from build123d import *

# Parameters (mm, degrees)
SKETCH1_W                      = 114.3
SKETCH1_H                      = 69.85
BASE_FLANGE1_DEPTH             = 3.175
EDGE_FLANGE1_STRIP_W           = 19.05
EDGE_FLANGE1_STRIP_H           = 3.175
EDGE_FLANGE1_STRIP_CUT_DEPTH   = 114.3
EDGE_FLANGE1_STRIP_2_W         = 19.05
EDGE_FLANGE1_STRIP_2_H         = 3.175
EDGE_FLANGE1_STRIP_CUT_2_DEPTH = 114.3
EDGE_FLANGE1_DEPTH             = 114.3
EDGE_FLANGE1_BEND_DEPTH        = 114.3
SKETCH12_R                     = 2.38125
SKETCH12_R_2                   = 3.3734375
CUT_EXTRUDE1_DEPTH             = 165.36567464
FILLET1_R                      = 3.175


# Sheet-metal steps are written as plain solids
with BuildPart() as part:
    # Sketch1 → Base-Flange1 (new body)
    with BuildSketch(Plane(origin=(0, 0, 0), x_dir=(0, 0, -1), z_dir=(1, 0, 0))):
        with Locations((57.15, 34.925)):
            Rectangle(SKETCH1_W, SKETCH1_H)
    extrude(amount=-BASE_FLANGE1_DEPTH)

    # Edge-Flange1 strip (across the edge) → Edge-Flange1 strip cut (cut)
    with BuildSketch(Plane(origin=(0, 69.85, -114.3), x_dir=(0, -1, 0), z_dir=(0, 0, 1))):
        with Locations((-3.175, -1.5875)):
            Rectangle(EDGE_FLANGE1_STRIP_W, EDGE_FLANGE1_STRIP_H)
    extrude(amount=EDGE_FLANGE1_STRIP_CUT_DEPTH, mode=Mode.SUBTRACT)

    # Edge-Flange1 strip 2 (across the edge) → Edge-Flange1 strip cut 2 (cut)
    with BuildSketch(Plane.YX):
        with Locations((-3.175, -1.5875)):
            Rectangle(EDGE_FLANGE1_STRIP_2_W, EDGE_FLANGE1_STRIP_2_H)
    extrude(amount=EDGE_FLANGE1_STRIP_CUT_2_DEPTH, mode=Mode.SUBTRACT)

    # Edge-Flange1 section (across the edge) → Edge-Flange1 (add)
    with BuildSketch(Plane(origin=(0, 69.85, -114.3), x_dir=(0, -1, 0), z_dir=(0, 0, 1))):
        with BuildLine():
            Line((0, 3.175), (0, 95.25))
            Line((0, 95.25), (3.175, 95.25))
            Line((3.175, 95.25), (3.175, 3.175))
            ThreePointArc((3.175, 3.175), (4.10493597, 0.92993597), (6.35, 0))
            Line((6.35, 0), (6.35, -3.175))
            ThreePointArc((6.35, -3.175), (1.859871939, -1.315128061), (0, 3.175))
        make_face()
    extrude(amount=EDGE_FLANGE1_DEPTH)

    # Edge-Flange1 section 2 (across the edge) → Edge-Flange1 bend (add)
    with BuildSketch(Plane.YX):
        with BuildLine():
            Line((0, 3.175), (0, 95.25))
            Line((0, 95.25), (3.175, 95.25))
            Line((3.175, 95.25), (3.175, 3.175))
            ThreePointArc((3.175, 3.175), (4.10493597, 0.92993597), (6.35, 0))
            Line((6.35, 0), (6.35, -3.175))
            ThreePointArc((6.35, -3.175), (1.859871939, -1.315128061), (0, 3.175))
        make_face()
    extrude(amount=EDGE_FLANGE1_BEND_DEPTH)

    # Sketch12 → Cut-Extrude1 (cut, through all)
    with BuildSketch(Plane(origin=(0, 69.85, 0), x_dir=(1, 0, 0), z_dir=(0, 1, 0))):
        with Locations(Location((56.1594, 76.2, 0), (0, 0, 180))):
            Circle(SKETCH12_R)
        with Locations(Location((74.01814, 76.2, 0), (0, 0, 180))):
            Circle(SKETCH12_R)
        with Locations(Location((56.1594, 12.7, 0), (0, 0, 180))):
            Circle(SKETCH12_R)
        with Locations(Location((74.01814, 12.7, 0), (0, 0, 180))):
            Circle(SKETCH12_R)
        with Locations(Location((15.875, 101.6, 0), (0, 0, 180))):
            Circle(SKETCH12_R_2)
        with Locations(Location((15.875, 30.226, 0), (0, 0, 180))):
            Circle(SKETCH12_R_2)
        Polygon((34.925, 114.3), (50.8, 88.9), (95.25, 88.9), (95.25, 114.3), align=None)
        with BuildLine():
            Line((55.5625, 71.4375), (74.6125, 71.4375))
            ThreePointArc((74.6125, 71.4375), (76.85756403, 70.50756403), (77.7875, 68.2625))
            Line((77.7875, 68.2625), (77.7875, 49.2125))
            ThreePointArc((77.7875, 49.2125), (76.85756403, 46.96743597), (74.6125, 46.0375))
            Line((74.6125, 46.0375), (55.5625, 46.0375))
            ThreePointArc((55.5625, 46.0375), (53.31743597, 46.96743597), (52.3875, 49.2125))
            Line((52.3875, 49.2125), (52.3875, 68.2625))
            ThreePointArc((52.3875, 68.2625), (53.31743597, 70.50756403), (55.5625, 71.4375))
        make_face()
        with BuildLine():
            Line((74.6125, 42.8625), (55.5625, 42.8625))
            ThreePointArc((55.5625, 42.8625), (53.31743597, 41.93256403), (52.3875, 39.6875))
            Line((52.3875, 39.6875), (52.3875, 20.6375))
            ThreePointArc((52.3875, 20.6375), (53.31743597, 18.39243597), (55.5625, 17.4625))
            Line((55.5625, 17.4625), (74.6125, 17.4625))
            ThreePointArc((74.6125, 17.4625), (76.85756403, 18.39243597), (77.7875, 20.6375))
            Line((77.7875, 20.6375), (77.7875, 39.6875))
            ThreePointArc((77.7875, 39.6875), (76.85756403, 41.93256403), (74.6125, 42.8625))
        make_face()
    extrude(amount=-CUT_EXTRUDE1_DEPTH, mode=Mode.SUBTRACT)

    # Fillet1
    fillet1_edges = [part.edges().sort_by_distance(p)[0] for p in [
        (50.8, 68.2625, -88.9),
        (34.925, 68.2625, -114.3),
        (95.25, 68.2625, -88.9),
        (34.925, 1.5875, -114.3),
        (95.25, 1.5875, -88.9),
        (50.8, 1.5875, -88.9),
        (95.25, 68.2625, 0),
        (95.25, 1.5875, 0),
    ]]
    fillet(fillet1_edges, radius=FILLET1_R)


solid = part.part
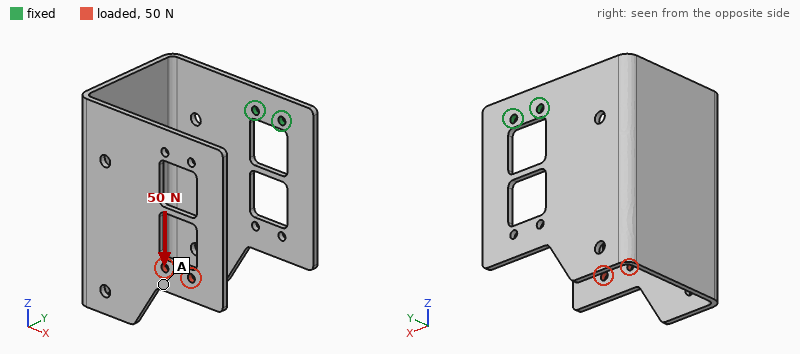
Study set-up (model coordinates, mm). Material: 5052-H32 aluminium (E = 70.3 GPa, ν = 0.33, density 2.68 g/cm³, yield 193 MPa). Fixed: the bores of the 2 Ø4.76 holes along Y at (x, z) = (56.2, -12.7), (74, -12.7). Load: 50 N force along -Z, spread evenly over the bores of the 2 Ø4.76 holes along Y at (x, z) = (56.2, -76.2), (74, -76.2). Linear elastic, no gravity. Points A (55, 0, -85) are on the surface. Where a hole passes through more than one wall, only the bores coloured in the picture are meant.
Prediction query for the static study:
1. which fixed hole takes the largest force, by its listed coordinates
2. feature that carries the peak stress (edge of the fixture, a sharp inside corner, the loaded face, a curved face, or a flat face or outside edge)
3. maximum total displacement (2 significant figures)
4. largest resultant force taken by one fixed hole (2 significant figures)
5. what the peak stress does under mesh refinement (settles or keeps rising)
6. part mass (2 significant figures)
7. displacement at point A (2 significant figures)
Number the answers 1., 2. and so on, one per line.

1. (56.2, -12.7)
2. edge of the fixture
3. 2.0 mm
4. 36 N
5. keeps rising
6. 200 g
7. 1.7 mm
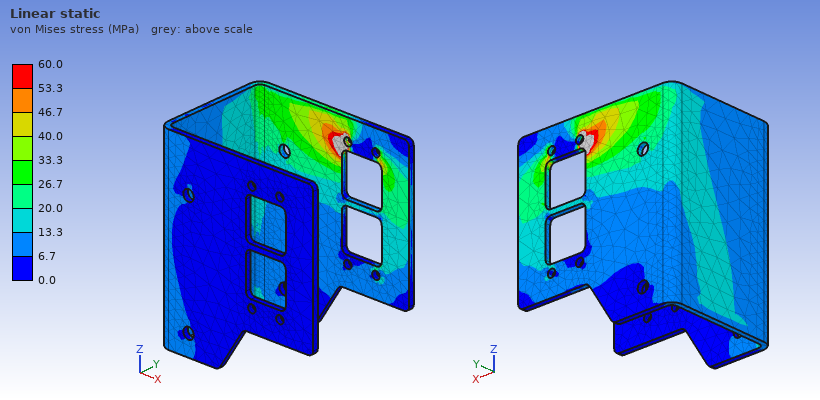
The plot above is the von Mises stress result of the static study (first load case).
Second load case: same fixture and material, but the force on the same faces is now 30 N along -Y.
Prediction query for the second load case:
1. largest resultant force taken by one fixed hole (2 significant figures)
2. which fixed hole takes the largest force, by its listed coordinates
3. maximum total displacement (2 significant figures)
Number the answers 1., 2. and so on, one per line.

1. 17 N
2. (74, -12.7)
3. 1.6 mm
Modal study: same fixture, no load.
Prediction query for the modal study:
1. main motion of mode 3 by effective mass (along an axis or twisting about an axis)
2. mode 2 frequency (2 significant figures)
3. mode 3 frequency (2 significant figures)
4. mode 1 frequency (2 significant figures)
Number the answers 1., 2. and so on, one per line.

1. along Y
2. 98 Hz
3. 190 Hz
4. 73 Hz
